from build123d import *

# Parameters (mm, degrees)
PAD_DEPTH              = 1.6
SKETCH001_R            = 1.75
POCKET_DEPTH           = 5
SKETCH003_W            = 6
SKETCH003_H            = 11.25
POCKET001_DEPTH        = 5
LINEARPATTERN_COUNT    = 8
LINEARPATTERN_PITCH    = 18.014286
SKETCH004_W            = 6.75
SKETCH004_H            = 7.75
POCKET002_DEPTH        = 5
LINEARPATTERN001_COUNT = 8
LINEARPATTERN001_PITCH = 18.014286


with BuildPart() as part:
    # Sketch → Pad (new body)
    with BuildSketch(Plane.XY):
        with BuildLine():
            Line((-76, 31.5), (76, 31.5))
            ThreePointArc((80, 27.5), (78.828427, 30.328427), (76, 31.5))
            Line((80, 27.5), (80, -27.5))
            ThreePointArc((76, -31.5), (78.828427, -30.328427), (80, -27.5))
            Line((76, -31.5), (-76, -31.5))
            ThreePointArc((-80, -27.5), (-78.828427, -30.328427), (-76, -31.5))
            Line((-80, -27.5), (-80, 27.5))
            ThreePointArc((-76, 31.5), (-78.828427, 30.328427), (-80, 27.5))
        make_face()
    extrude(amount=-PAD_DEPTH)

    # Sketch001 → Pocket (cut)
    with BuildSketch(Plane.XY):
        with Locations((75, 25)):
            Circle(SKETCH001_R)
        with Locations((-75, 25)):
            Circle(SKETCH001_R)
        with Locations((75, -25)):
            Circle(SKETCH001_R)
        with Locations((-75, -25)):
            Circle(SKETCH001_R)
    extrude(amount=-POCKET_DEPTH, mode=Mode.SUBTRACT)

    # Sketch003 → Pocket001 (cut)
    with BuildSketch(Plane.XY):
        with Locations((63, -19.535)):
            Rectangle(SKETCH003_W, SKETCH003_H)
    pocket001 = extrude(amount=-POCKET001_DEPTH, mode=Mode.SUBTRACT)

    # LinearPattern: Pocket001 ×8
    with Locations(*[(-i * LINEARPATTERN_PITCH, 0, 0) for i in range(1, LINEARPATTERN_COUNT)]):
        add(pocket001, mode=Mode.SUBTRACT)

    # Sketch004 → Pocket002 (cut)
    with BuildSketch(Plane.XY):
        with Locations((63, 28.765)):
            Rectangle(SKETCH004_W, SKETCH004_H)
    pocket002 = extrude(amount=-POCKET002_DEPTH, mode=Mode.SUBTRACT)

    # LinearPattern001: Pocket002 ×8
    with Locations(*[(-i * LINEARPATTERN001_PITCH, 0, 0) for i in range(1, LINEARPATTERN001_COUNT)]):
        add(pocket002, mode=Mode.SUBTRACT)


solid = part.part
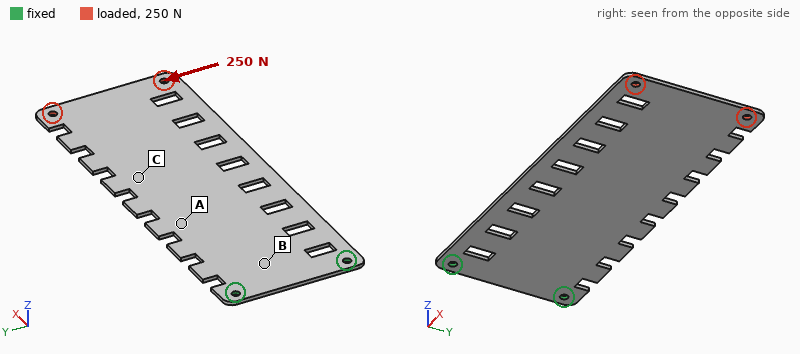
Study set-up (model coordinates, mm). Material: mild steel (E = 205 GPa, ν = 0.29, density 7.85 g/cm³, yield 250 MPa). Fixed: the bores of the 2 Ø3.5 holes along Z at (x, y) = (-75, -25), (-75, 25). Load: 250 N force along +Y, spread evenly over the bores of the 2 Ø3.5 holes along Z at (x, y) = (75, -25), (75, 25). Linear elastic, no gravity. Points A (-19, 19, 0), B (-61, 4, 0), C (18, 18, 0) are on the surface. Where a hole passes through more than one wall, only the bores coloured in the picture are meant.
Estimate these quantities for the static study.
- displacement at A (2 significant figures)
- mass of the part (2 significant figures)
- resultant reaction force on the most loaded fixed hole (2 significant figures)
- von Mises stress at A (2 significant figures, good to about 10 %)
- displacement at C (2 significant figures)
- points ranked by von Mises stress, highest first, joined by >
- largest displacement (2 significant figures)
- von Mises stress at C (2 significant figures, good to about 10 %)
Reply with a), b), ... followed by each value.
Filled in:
a) 20 µm
b) 110 g
c) 780 N
d) 25 MPa
e) 42 µm
f) A > C > B
g) 91 µm
h) 14 MPa
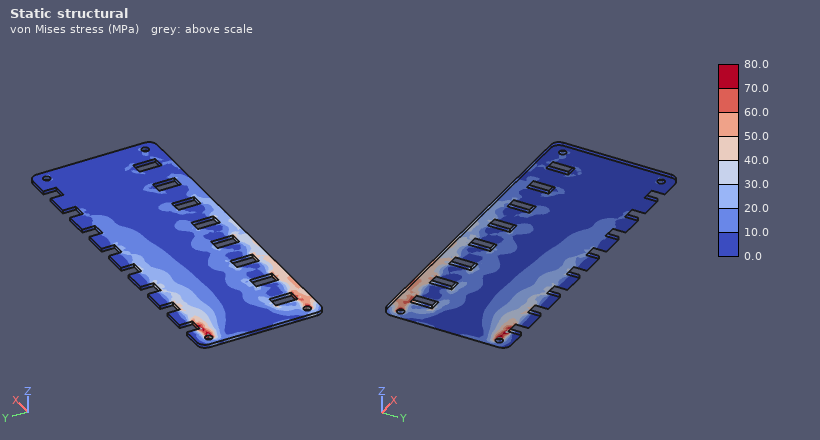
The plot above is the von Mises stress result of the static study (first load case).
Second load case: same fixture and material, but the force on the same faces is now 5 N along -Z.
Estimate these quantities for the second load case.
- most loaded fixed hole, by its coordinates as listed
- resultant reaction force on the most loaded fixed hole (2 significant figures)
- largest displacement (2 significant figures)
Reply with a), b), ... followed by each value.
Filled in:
a) (-75, -25)
b) 2.7 N
c) 1.9 mm
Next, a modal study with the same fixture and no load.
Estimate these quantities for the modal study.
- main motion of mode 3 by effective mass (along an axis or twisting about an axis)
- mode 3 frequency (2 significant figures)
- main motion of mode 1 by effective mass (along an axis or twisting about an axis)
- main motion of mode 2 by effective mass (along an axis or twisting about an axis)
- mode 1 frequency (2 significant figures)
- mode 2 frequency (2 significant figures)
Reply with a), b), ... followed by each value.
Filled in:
a) along Z
b) 310 Hz
c) along Z
d) twisting about X
e) 48 Hz
f) 280 Hz
